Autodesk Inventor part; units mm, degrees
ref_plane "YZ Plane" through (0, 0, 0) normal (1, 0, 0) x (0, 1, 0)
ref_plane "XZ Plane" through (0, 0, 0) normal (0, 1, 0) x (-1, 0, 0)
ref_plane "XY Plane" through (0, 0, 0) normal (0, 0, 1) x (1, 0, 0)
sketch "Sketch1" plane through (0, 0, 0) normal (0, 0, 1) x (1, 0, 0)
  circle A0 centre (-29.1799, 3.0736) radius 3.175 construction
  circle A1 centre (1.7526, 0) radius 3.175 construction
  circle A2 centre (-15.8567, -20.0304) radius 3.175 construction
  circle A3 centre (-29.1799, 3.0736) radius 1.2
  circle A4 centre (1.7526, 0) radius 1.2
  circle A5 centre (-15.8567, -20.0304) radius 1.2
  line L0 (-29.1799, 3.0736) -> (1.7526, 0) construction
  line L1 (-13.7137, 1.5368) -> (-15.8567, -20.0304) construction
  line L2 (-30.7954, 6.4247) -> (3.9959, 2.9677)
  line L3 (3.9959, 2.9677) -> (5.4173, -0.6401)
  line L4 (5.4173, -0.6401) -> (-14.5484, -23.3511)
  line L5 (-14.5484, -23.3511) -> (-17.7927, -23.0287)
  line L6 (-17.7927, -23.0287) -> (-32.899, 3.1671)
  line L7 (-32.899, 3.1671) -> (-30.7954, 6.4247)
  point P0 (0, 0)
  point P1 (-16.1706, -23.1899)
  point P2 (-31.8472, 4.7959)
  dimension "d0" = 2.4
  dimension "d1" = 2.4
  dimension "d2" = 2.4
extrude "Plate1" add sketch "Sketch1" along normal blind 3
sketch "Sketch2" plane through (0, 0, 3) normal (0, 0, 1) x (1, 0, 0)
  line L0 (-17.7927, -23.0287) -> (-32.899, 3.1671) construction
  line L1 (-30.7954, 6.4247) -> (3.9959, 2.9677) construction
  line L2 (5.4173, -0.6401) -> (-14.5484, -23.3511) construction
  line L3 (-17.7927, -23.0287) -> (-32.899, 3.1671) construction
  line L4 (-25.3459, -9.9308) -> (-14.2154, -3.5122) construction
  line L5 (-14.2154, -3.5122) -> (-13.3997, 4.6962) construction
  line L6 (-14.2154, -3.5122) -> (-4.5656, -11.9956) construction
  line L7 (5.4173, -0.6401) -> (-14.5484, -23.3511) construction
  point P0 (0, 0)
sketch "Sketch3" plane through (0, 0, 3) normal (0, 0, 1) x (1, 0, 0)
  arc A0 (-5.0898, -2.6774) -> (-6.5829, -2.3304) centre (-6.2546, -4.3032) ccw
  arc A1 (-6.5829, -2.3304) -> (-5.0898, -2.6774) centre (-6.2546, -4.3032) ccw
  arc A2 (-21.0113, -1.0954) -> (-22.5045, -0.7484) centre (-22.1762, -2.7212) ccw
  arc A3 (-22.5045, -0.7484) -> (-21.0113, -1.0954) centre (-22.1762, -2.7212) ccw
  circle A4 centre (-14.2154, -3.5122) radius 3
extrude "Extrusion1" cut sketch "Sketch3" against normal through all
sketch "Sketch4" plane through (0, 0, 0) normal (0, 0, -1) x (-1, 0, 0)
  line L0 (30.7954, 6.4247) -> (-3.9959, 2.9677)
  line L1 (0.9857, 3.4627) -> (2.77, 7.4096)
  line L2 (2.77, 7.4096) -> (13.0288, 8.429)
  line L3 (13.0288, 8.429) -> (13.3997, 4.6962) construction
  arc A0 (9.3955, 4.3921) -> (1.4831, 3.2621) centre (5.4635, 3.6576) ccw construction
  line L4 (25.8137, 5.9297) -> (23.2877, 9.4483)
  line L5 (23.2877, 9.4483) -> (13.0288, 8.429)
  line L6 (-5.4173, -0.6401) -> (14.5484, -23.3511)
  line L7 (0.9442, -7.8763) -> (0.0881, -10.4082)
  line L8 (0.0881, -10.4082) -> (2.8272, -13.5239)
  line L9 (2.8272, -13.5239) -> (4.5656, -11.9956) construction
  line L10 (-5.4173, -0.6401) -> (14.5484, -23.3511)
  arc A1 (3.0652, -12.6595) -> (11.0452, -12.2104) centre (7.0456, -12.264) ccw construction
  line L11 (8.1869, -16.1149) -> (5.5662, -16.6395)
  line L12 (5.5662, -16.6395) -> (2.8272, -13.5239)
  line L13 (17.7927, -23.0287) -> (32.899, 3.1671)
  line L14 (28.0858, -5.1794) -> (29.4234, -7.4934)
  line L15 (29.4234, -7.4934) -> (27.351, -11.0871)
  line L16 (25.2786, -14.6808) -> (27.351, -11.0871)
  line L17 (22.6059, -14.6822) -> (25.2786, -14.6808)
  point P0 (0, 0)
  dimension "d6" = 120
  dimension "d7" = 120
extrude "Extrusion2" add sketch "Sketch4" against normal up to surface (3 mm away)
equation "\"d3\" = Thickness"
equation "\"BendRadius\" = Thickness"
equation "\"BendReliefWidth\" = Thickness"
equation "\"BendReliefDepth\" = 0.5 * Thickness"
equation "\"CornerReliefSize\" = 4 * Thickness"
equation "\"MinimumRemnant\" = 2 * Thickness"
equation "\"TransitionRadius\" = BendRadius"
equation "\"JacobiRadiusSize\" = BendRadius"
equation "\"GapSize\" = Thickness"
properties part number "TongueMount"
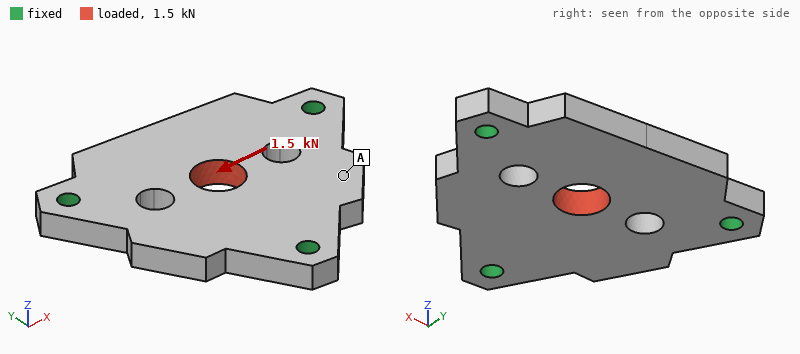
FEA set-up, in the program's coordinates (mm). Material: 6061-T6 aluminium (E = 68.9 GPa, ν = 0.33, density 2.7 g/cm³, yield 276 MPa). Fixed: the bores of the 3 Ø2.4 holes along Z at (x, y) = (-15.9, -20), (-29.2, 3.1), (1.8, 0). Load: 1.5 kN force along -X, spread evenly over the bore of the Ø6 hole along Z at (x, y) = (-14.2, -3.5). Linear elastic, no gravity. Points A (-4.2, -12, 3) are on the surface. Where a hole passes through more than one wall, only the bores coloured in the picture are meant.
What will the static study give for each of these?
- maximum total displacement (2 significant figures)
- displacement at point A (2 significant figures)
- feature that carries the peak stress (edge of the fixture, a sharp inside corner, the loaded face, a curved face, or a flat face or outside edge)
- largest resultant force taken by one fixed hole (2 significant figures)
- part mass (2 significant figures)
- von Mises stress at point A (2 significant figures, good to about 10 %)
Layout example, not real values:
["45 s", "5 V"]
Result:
["8.6 µm", "5.4 µm", "a curved face", "610 N", "5.7 g", "10 MPa"]
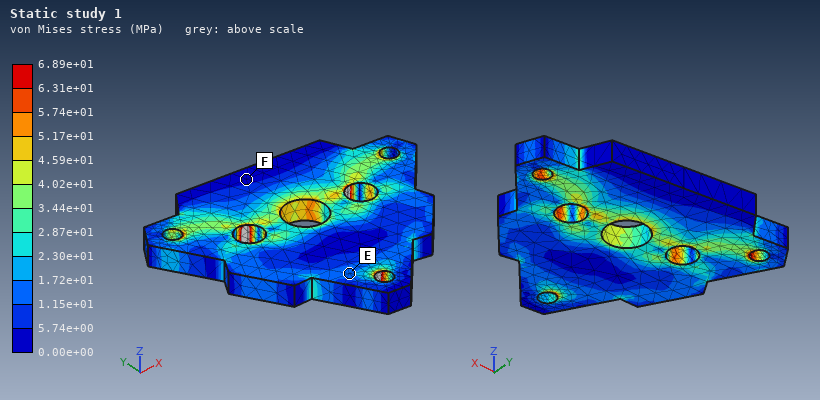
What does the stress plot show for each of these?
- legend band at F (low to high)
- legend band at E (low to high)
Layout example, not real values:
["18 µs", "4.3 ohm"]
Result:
["0.00e+00 to 5.74e+00 MPa", "1.15e+01 to 1.72e+01 MPa"]
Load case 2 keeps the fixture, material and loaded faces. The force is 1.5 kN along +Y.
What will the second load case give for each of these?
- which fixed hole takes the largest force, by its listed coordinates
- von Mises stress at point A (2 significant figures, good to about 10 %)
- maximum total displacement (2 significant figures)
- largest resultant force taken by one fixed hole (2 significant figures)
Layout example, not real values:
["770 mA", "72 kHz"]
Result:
["(-15.9, -20)", "8.5 MPa", "9.9 µm", "790 N"]
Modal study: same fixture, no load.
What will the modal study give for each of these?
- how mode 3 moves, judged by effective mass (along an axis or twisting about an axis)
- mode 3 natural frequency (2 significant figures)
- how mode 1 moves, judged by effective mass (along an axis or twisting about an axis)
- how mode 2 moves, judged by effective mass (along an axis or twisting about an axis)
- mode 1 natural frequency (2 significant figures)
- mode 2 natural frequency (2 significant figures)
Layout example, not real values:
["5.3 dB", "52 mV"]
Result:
["twisting about Y", "20 kHz", "along Z", "along Z", "14 kHz", "19 kHz"]
